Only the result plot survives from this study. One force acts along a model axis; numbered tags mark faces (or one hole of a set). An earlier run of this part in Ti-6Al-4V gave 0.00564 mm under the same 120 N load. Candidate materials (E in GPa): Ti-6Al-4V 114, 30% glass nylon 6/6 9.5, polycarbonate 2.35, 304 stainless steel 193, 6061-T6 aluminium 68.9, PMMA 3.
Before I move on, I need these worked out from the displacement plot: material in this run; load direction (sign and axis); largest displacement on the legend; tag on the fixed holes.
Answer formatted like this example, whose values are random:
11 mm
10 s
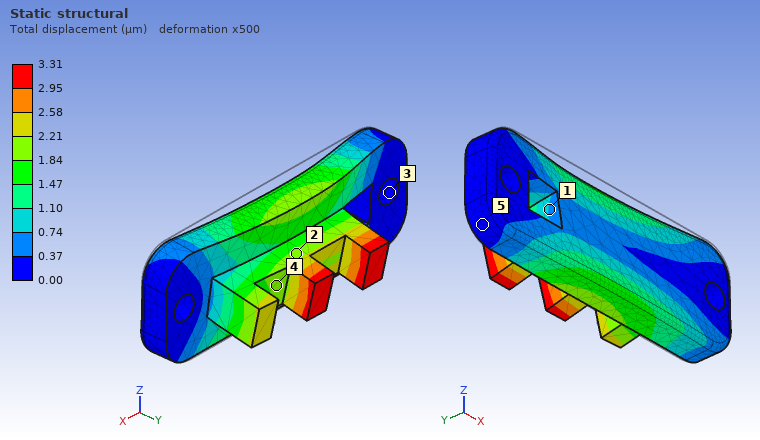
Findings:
304 stainless steel
-Z
3.31 µm
3
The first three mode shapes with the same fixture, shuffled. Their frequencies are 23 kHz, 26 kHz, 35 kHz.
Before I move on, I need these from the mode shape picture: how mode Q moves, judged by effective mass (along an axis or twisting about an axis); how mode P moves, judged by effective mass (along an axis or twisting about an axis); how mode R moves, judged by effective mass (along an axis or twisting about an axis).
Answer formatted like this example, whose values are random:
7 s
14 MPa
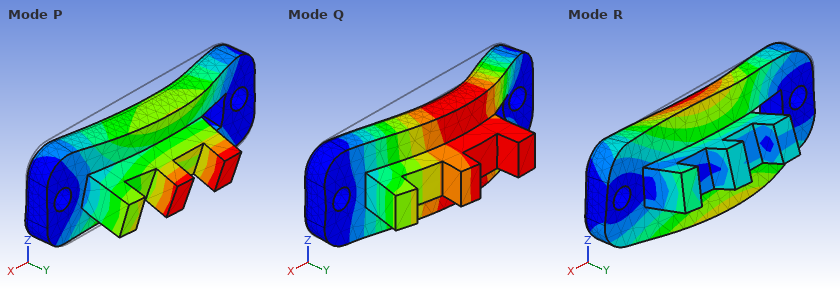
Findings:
along Y
along Z
along Z
